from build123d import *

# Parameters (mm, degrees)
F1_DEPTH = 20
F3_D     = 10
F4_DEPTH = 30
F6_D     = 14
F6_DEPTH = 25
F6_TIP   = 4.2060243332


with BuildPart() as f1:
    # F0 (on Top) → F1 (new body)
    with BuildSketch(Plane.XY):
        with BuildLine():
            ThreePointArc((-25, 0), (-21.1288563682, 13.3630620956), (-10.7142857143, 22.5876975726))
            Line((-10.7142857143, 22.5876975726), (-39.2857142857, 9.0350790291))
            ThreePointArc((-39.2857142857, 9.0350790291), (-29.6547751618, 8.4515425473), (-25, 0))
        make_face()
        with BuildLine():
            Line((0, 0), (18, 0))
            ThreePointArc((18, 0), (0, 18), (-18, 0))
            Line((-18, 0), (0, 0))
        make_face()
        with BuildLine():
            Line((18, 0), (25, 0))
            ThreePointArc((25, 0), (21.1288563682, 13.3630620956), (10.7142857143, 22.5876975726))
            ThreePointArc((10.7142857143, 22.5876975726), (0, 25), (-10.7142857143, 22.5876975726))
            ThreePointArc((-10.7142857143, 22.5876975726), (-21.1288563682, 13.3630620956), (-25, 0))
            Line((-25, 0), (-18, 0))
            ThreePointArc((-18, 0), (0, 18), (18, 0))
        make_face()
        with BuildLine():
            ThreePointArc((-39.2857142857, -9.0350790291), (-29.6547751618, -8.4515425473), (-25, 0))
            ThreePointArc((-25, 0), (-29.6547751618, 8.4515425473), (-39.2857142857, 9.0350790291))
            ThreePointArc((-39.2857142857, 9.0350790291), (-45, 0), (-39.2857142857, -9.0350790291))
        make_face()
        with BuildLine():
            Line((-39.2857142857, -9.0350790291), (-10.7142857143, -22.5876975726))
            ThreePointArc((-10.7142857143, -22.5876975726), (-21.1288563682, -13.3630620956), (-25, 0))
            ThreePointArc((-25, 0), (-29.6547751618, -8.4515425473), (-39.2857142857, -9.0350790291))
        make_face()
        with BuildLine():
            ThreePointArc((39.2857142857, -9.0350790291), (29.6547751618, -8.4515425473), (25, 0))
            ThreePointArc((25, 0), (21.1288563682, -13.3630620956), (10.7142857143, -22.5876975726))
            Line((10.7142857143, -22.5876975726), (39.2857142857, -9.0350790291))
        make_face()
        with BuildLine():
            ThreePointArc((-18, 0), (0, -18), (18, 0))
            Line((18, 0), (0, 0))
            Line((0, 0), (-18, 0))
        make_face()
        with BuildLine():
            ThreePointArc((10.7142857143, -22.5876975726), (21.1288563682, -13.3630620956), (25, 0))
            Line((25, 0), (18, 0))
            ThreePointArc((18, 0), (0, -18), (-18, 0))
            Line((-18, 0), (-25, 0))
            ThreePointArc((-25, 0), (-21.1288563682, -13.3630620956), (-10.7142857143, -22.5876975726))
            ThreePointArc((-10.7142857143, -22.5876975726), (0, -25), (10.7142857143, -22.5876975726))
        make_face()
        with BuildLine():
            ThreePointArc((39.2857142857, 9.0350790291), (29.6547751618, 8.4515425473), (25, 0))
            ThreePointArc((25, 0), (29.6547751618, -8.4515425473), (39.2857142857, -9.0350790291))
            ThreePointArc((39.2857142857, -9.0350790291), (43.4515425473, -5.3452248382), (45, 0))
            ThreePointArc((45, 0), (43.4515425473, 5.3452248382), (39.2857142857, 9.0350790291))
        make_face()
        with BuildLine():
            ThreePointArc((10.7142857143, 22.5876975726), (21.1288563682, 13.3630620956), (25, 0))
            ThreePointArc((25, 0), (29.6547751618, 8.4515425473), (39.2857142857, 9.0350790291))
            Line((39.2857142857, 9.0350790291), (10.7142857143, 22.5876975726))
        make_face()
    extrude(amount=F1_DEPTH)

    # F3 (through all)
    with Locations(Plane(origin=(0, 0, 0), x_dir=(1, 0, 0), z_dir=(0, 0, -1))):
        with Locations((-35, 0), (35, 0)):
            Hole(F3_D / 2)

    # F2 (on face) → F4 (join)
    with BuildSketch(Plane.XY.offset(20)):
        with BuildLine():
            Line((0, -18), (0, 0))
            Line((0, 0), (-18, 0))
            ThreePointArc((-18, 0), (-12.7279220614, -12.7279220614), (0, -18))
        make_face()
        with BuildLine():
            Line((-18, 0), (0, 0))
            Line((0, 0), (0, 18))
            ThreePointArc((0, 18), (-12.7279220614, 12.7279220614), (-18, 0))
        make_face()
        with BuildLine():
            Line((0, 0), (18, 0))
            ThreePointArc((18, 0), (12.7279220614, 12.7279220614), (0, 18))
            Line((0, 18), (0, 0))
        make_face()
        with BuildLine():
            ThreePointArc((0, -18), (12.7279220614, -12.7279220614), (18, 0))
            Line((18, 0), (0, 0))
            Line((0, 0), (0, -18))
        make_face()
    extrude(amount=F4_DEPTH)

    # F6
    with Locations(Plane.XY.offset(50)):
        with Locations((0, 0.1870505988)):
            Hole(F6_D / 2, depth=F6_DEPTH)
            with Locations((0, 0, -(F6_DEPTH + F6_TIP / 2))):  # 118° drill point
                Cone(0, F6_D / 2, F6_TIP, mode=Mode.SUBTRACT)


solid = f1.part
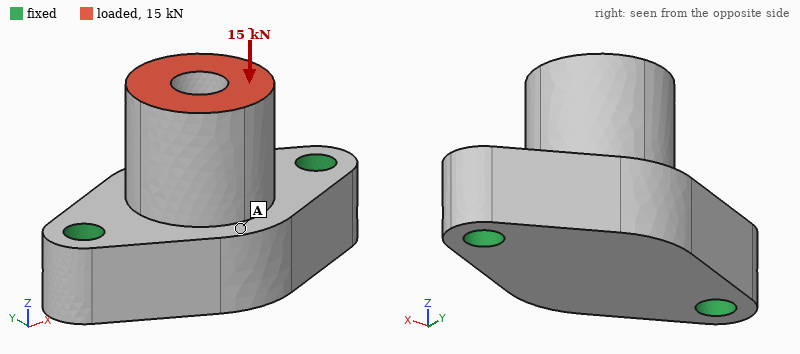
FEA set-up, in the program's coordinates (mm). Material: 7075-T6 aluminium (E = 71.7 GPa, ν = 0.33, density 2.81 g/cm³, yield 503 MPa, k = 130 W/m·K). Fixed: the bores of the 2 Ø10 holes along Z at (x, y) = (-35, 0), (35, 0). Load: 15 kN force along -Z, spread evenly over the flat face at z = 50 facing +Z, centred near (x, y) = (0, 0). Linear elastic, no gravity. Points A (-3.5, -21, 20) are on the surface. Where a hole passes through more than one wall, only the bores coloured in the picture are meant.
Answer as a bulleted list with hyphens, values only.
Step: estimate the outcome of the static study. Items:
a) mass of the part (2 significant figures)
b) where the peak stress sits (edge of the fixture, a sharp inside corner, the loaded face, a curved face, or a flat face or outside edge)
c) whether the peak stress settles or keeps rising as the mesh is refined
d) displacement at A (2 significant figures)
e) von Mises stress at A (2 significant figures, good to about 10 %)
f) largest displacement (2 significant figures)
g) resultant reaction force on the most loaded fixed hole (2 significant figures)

- 230 g
- edge of the fixture
- keeps rising
- 19 µm
- 13 MPa
- 25 µm
- 7.6 kN
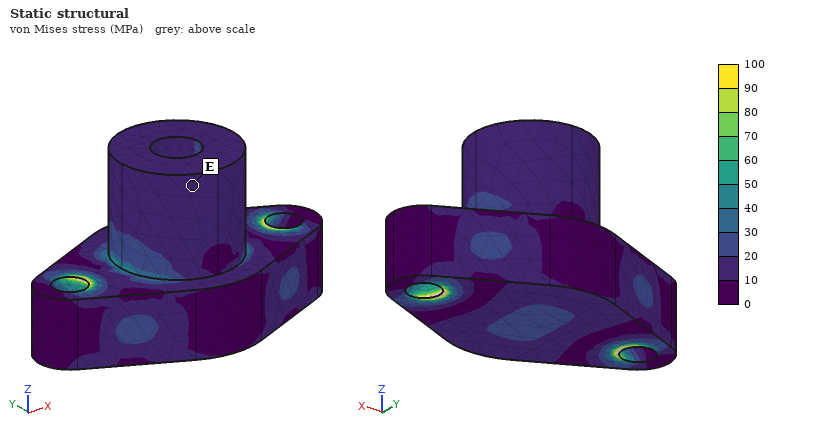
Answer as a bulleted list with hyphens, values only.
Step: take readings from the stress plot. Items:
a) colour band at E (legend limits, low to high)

- 10 to 20 MPa
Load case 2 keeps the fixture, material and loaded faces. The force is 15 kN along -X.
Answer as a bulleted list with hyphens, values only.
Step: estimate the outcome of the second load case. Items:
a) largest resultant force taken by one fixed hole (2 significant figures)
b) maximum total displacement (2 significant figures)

- 13 kN
- 0.11 mm
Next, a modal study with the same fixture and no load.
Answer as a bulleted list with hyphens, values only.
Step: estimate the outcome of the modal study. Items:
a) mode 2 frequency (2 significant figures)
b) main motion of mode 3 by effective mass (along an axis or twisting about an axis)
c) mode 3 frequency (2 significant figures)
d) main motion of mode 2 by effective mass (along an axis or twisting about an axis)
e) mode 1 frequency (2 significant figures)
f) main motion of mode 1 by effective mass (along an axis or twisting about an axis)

- 11 kHz
- along X
- 11 kHz
- along Z
- 6000 Hz
- along Y
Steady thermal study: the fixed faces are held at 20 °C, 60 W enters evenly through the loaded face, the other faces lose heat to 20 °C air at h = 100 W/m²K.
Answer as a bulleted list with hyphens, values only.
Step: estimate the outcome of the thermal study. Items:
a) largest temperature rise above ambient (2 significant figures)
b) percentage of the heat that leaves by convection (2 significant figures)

- 23 K
- 18 %
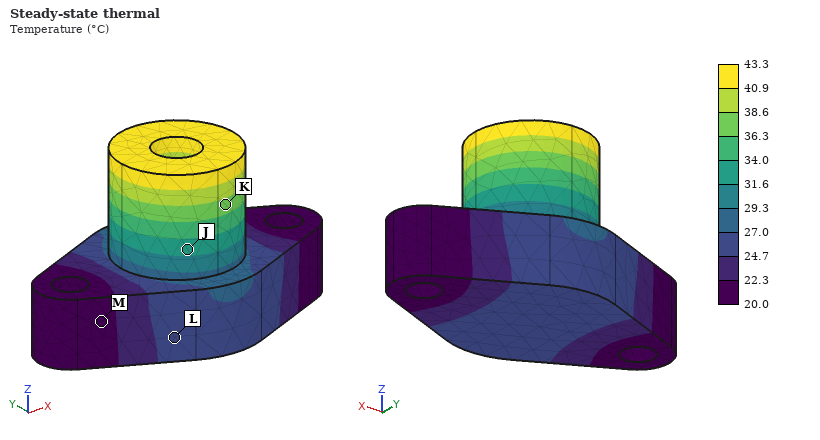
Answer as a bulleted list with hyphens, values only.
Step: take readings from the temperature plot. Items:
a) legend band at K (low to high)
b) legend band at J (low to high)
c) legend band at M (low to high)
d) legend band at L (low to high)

- 36.3 to 38.6 °C
- 31.6 to 34.0 °C
- 20.0 to 22.3 °C
- 24.7 to 27.0 °C
